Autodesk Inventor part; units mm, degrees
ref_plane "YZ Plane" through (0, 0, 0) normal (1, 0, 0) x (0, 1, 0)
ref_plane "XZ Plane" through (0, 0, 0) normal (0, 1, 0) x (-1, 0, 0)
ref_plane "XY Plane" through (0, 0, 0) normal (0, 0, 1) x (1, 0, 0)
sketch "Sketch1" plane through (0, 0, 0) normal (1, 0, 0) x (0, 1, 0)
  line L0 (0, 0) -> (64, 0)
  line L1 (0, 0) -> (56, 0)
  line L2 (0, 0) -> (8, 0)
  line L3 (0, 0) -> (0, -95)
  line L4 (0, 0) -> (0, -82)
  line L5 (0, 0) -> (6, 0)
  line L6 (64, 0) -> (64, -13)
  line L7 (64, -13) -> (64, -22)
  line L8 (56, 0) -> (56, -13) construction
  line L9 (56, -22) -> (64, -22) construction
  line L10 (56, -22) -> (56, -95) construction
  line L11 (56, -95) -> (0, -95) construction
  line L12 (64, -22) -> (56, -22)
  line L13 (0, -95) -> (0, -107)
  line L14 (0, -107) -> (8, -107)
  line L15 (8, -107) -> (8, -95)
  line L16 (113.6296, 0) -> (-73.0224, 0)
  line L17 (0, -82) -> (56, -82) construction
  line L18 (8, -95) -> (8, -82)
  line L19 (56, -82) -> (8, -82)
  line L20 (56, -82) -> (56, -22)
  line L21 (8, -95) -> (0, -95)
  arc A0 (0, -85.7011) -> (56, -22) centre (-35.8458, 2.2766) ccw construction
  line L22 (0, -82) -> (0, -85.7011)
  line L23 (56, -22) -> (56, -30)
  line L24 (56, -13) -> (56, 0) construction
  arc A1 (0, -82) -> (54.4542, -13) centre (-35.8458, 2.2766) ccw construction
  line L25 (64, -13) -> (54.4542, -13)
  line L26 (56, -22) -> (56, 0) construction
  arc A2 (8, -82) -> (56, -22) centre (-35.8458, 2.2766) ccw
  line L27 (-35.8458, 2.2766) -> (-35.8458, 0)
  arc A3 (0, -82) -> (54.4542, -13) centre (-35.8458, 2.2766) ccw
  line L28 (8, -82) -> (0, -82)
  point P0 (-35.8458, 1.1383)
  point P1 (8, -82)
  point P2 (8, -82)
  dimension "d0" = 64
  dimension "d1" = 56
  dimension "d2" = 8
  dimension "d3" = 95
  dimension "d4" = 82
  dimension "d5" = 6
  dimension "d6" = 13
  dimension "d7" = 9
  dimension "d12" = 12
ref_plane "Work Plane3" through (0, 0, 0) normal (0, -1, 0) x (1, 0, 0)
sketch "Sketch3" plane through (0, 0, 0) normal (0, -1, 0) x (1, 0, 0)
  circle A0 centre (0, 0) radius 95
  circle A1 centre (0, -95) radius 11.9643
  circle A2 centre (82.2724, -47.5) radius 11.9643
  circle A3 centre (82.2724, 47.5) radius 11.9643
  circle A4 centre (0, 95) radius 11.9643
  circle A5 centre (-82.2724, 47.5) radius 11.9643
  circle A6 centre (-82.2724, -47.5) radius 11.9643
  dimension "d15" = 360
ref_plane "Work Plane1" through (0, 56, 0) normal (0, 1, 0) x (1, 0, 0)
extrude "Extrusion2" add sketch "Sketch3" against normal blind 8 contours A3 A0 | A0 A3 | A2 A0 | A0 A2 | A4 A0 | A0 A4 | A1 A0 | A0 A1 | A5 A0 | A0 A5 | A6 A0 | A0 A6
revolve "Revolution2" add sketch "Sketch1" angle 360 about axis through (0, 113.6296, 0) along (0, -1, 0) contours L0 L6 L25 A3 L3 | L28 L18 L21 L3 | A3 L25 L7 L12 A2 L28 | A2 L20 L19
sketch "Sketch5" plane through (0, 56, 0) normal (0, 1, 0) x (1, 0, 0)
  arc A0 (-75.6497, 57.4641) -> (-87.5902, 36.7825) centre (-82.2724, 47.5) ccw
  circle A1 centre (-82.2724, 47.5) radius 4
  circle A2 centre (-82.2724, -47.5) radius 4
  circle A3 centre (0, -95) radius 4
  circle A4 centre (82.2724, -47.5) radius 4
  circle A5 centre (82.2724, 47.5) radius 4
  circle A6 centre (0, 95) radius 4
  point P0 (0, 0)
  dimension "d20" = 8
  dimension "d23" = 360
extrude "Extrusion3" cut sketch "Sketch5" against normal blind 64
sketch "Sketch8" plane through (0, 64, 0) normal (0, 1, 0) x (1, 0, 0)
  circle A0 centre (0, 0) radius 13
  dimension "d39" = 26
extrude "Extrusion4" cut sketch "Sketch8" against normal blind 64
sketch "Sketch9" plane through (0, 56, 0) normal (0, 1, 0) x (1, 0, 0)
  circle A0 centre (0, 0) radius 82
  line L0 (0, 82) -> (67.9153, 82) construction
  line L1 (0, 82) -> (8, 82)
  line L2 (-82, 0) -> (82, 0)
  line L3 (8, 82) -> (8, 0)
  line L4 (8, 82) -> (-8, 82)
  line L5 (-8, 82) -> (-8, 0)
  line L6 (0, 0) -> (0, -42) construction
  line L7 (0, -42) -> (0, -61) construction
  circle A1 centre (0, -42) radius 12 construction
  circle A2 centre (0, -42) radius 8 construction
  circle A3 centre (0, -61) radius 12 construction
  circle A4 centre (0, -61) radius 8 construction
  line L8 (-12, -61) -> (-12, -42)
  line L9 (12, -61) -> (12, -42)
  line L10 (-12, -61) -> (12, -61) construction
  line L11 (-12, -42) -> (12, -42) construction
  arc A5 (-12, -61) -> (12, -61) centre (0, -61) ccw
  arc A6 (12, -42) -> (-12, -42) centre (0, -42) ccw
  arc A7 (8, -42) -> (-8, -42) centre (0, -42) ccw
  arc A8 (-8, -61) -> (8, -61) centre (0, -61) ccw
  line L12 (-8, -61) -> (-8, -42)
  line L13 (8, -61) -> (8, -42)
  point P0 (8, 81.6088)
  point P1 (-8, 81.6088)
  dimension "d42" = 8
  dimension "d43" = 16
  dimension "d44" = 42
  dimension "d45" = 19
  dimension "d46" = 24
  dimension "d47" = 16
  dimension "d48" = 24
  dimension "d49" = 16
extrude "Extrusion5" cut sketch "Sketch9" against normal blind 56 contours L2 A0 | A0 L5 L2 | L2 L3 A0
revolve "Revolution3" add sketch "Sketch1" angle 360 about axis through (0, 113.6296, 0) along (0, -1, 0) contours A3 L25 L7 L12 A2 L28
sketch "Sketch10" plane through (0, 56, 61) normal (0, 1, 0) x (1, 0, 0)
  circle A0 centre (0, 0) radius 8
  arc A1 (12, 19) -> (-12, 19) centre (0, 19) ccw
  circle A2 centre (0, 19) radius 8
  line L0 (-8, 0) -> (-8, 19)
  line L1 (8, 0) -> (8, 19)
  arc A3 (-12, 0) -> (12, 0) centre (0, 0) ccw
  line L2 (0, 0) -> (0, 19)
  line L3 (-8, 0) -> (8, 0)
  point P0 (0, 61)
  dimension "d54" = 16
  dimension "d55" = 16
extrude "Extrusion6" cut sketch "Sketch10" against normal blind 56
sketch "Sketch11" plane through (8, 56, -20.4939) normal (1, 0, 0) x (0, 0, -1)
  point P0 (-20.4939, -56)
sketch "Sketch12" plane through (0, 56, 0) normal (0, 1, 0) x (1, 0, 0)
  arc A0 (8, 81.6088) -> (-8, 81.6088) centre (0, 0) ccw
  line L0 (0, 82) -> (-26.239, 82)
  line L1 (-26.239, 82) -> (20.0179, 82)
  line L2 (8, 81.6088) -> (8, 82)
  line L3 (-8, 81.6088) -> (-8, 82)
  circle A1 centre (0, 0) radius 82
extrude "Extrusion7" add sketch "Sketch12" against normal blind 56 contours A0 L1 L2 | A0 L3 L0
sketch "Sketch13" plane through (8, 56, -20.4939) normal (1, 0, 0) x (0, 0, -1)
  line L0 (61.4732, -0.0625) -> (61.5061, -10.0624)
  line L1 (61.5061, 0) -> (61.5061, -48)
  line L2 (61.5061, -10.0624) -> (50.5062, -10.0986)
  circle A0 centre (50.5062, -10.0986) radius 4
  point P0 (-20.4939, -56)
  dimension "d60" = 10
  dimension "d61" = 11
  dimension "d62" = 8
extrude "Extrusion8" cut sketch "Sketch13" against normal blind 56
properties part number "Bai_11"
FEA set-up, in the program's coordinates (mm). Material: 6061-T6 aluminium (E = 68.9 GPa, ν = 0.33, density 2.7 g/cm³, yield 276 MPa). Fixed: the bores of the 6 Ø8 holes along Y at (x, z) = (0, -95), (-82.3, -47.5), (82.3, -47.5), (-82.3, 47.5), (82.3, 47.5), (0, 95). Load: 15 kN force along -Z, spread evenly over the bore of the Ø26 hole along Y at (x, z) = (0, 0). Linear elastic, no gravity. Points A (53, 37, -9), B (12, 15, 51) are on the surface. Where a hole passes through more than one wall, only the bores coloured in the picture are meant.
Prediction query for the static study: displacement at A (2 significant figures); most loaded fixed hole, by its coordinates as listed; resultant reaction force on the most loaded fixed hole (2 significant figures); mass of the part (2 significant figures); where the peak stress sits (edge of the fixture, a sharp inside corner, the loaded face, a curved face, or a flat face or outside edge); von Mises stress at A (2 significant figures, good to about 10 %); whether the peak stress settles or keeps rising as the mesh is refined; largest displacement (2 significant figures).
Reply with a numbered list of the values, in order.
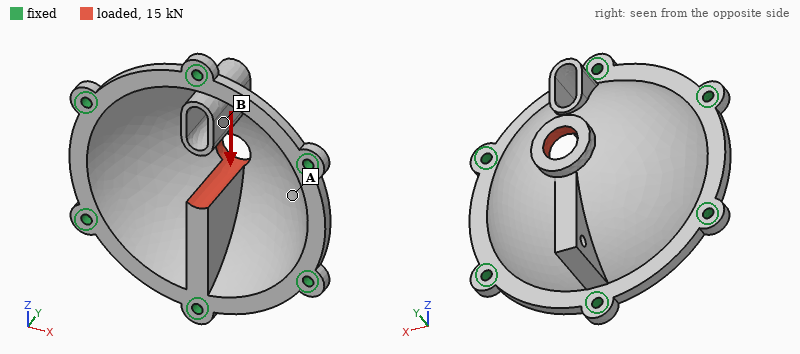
1. 21 µm
2. (0, -95)
3. 7.8 kN
4. 670 g
5. edge of the fixture
6. 17 MPa
7. keeps rising
8. 57 µm
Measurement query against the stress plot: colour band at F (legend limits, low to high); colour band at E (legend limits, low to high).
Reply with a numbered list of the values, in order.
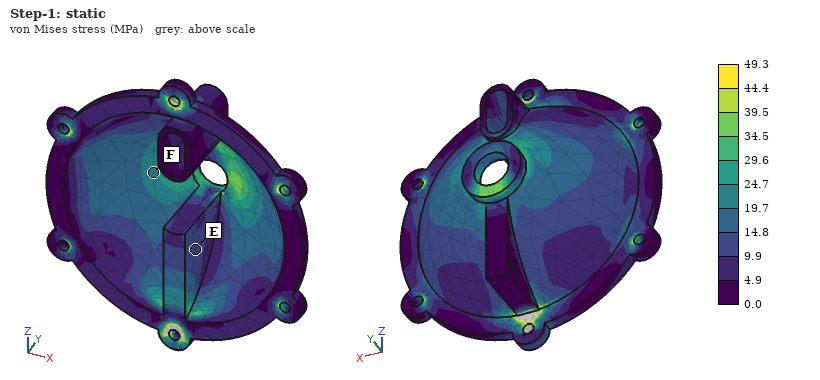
1. 19.7 to 24.7 MPa
2. 9.9 to 14.8 MPa
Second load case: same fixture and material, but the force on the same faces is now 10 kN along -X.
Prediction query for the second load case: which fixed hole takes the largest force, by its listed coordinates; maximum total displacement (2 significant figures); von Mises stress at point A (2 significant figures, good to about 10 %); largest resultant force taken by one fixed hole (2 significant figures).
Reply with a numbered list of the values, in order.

1. (0, -95)
2. 0.43 mm
3. 13 MPa
4. 4.0 kN
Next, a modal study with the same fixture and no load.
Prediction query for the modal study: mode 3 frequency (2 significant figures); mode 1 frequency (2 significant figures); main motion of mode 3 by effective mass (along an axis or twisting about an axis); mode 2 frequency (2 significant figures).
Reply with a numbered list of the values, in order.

1. 4000 Hz
2. 2900 Hz
3. along Y
4. 3700 Hz
